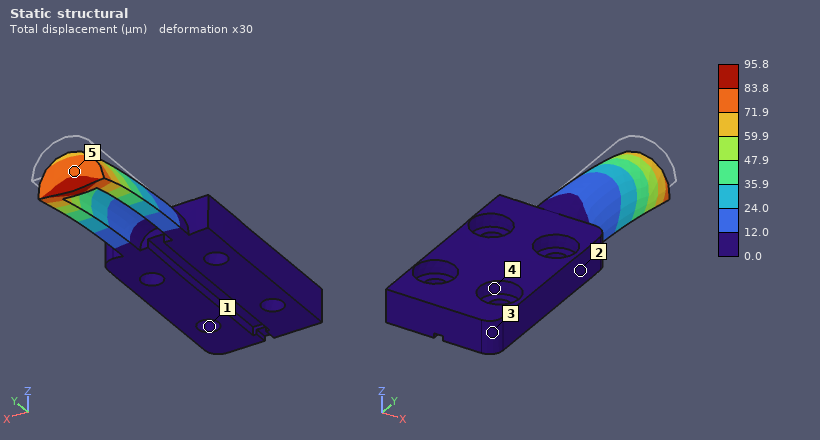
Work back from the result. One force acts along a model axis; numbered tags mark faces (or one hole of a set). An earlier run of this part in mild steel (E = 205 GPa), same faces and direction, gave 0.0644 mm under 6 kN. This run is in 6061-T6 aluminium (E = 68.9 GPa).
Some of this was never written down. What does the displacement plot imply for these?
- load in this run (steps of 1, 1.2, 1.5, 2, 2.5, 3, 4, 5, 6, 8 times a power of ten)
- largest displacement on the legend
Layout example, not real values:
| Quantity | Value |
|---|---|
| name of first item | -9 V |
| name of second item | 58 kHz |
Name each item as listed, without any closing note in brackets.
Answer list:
| Quantity | Value |
|---|---|
| load in this run | 3 kN |
| largest displacement on the legend | 95.8 µm |
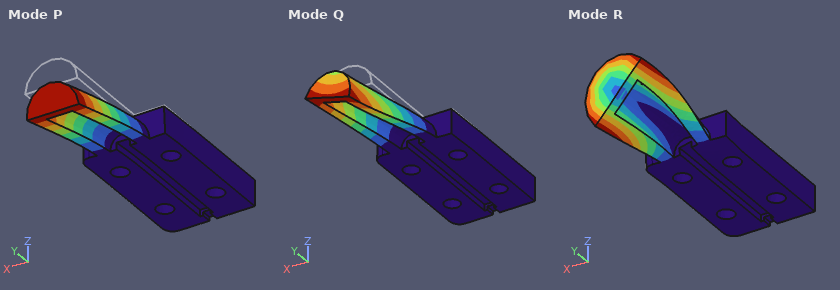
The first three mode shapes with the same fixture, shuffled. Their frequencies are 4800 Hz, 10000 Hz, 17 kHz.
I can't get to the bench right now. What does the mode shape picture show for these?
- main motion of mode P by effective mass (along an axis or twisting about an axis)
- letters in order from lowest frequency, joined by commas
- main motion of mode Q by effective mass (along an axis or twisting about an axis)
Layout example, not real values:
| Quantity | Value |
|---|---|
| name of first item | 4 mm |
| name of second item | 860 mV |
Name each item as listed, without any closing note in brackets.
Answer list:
| Quantity | Value |
|---|---|
| main motion of mode P by effective mass | along Z |
| letters in order from lowest frequency, joined by commas | P, Q, R |
| main motion of mode Q by effective mass | along X |
